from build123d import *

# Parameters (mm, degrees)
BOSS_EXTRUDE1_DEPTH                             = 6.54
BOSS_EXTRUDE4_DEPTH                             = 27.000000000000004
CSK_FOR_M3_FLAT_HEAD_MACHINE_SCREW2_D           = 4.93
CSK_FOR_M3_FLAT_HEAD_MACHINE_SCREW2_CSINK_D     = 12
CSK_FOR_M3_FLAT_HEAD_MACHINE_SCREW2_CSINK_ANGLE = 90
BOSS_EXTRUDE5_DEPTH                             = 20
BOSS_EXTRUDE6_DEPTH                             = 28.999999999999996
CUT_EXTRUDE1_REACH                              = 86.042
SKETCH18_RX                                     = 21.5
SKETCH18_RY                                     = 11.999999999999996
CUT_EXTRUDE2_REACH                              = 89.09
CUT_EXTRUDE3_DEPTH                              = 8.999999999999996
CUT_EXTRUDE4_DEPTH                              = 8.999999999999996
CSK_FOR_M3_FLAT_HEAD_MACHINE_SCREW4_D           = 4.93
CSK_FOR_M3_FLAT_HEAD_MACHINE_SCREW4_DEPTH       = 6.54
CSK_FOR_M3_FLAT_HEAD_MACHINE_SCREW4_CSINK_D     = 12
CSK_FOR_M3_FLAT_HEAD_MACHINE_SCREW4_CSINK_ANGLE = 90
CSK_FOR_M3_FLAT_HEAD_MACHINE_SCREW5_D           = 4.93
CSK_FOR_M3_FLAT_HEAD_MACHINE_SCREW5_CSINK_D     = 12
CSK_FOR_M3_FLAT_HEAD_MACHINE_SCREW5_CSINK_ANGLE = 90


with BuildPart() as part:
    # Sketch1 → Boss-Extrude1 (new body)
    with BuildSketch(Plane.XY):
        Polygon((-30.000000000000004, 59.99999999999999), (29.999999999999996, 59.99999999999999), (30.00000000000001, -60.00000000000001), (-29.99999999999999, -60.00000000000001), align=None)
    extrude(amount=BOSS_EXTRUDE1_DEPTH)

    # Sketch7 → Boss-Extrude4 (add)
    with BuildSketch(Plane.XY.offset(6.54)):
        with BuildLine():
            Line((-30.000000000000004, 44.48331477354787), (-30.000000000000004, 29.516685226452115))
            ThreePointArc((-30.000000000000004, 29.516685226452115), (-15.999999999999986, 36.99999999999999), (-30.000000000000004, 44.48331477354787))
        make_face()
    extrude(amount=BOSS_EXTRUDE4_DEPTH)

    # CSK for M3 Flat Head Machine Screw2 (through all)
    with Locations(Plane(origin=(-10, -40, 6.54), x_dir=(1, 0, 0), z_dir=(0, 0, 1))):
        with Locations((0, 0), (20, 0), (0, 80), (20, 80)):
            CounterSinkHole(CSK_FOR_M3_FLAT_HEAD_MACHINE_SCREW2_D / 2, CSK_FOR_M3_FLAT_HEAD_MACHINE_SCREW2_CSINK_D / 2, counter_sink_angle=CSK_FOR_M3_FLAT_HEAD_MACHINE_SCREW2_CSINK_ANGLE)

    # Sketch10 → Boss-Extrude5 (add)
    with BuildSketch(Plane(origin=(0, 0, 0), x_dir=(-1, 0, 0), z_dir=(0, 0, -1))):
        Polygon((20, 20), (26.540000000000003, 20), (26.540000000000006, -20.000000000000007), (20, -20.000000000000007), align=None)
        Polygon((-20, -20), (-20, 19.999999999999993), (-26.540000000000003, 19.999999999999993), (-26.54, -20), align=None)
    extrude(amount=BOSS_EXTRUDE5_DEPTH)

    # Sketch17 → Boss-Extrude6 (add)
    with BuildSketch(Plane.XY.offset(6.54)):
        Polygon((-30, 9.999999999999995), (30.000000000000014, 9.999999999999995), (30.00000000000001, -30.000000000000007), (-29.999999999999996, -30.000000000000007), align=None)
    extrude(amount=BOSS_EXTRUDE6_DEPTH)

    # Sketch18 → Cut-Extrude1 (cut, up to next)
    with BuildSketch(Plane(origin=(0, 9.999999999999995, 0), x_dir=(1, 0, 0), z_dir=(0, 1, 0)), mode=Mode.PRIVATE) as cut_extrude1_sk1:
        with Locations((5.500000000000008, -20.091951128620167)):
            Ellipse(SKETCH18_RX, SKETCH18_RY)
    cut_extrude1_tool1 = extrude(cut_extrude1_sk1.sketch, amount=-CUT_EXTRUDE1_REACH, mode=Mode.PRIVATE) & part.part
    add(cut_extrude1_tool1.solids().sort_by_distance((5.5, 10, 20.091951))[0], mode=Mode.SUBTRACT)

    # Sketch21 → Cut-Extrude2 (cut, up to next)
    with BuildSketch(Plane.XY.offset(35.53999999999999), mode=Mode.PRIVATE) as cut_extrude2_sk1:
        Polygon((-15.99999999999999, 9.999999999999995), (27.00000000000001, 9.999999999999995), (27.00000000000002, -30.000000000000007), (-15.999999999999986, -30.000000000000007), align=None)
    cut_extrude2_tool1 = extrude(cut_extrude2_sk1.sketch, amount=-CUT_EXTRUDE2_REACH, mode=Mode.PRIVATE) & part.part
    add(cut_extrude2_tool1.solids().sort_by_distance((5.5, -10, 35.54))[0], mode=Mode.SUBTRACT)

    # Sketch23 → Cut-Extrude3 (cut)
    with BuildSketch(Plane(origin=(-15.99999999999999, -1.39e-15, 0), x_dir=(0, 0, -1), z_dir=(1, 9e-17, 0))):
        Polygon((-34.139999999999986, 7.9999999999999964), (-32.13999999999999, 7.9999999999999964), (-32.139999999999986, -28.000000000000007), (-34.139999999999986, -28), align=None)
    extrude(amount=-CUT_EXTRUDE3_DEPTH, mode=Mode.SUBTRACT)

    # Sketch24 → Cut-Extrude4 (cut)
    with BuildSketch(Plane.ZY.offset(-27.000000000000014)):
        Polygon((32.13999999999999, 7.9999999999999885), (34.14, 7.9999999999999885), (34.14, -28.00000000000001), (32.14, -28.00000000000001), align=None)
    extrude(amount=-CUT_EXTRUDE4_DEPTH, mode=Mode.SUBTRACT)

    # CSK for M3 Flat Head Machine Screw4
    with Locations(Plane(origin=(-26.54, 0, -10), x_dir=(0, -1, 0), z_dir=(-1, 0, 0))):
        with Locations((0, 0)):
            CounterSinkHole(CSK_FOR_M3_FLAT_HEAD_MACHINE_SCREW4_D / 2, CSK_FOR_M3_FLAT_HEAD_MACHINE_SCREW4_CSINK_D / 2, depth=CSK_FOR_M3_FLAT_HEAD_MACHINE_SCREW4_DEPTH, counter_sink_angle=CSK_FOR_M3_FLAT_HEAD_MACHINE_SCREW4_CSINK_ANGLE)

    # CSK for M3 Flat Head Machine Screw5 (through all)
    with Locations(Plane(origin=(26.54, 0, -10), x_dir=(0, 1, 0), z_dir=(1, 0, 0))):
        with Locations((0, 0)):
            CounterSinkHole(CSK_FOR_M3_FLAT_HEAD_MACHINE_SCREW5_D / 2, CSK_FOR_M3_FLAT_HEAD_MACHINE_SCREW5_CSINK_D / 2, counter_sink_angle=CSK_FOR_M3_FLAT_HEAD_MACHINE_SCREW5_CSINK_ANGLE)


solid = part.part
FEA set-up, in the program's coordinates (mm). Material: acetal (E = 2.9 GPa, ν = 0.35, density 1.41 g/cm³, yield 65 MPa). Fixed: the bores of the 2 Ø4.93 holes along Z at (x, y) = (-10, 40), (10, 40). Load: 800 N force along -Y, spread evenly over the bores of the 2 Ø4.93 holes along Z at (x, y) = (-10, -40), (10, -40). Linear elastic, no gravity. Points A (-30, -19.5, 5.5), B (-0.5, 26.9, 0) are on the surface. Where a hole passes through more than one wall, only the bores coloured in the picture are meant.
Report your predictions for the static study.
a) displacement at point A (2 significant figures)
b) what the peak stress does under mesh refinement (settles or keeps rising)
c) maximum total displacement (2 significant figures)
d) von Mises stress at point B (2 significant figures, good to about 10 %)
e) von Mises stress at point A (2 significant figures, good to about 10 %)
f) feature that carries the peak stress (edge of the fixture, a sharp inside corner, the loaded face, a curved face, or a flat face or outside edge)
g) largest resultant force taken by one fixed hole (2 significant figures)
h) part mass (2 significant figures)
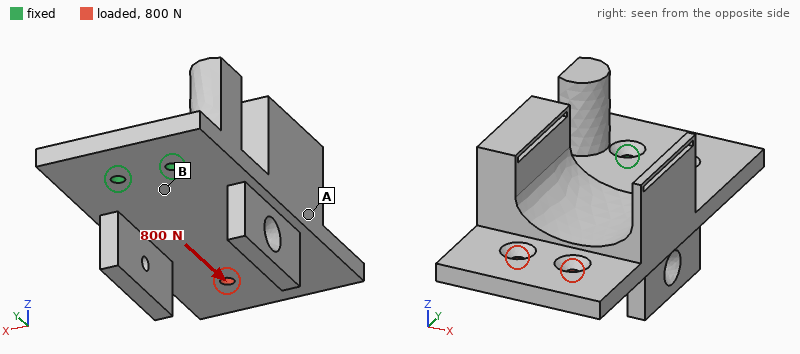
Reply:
0.36 mm
keeps rising
0.91 mm
4.9 MPa
1.1 MPa
edge of the fixture
400 N
120 g
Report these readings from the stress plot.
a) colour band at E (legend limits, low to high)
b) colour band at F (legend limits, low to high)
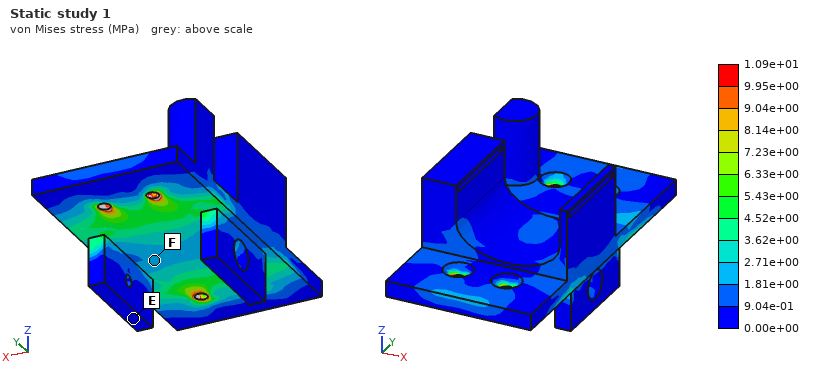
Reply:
0.00e+00 to 9.04e-01 MPa
1.81e+00 to 2.71e+00 MPa
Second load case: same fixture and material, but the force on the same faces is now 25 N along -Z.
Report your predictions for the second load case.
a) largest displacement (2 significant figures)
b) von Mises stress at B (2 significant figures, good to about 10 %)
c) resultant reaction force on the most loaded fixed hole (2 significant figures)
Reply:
1.5 mm
3.3 MPa
14 N
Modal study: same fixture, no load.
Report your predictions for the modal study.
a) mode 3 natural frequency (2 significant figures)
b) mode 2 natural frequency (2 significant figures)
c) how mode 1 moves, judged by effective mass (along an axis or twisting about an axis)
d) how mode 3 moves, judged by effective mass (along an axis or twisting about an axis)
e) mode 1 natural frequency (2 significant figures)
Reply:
530 Hz
370 Hz
along Z
along X
110 Hz
